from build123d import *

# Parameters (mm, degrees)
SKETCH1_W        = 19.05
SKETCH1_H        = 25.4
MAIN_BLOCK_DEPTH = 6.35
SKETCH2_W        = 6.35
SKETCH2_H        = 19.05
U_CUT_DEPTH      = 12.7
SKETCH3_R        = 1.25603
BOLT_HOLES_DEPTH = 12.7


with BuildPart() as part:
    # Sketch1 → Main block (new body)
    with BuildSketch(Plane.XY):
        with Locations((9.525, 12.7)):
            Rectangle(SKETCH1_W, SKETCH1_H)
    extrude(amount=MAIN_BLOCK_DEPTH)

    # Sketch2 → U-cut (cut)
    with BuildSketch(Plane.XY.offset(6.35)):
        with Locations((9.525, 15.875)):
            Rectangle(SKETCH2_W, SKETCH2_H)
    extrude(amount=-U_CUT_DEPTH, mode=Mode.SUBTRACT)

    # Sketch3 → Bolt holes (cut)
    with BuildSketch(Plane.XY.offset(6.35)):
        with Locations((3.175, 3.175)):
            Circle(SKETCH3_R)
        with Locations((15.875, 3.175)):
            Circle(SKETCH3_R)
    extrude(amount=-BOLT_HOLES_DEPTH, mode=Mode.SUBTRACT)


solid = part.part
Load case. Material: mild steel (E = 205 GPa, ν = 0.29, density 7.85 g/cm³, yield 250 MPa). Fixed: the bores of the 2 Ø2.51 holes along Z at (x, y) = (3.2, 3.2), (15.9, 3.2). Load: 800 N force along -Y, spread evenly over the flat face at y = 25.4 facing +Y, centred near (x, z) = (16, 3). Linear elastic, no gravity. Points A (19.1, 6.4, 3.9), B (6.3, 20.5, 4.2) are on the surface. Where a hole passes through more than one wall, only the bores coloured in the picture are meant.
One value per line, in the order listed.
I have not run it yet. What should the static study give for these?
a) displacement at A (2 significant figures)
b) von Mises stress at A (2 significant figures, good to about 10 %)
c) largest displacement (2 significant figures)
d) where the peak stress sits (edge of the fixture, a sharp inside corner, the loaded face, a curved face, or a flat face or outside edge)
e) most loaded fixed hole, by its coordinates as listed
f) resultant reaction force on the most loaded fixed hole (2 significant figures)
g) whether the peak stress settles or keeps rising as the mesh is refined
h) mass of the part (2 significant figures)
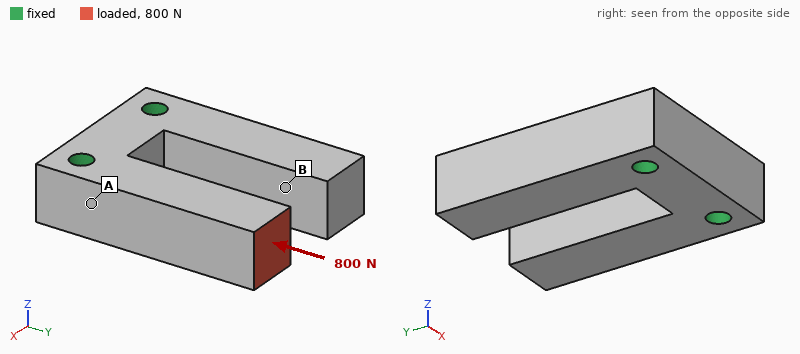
0.43 µm
16 MPa
2.3 µm
edge of the fixture
(15.9, 3.2)
780 N
keeps rising
18 g
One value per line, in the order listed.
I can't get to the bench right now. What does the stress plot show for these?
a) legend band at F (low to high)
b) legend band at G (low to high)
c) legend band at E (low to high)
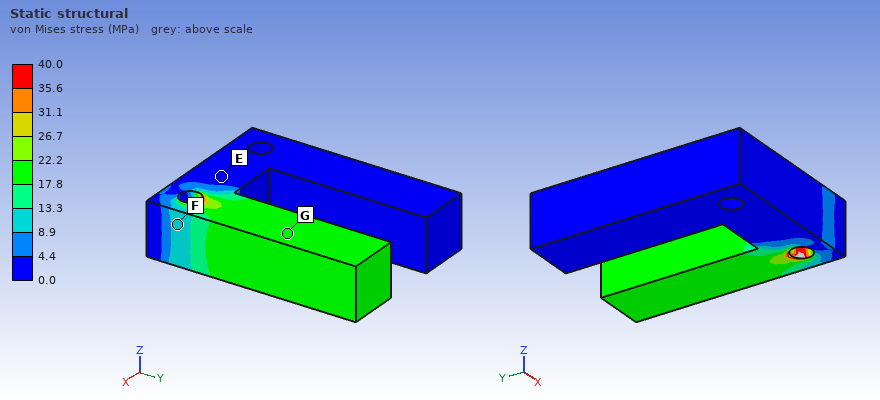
8.9 to 13.3 MPa
17.8 to 22.2 MPa
0.0 to 4.4 MPa
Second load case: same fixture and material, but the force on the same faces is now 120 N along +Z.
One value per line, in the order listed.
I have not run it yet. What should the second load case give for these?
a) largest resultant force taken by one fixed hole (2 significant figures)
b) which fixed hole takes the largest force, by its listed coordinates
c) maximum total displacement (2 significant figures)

130 N
(15.9, 3.2)
16 µm
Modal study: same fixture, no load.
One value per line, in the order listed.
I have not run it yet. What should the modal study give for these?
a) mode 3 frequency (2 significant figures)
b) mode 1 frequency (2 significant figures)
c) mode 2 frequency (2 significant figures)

10 kHz
9900 Hz
10 kHz
